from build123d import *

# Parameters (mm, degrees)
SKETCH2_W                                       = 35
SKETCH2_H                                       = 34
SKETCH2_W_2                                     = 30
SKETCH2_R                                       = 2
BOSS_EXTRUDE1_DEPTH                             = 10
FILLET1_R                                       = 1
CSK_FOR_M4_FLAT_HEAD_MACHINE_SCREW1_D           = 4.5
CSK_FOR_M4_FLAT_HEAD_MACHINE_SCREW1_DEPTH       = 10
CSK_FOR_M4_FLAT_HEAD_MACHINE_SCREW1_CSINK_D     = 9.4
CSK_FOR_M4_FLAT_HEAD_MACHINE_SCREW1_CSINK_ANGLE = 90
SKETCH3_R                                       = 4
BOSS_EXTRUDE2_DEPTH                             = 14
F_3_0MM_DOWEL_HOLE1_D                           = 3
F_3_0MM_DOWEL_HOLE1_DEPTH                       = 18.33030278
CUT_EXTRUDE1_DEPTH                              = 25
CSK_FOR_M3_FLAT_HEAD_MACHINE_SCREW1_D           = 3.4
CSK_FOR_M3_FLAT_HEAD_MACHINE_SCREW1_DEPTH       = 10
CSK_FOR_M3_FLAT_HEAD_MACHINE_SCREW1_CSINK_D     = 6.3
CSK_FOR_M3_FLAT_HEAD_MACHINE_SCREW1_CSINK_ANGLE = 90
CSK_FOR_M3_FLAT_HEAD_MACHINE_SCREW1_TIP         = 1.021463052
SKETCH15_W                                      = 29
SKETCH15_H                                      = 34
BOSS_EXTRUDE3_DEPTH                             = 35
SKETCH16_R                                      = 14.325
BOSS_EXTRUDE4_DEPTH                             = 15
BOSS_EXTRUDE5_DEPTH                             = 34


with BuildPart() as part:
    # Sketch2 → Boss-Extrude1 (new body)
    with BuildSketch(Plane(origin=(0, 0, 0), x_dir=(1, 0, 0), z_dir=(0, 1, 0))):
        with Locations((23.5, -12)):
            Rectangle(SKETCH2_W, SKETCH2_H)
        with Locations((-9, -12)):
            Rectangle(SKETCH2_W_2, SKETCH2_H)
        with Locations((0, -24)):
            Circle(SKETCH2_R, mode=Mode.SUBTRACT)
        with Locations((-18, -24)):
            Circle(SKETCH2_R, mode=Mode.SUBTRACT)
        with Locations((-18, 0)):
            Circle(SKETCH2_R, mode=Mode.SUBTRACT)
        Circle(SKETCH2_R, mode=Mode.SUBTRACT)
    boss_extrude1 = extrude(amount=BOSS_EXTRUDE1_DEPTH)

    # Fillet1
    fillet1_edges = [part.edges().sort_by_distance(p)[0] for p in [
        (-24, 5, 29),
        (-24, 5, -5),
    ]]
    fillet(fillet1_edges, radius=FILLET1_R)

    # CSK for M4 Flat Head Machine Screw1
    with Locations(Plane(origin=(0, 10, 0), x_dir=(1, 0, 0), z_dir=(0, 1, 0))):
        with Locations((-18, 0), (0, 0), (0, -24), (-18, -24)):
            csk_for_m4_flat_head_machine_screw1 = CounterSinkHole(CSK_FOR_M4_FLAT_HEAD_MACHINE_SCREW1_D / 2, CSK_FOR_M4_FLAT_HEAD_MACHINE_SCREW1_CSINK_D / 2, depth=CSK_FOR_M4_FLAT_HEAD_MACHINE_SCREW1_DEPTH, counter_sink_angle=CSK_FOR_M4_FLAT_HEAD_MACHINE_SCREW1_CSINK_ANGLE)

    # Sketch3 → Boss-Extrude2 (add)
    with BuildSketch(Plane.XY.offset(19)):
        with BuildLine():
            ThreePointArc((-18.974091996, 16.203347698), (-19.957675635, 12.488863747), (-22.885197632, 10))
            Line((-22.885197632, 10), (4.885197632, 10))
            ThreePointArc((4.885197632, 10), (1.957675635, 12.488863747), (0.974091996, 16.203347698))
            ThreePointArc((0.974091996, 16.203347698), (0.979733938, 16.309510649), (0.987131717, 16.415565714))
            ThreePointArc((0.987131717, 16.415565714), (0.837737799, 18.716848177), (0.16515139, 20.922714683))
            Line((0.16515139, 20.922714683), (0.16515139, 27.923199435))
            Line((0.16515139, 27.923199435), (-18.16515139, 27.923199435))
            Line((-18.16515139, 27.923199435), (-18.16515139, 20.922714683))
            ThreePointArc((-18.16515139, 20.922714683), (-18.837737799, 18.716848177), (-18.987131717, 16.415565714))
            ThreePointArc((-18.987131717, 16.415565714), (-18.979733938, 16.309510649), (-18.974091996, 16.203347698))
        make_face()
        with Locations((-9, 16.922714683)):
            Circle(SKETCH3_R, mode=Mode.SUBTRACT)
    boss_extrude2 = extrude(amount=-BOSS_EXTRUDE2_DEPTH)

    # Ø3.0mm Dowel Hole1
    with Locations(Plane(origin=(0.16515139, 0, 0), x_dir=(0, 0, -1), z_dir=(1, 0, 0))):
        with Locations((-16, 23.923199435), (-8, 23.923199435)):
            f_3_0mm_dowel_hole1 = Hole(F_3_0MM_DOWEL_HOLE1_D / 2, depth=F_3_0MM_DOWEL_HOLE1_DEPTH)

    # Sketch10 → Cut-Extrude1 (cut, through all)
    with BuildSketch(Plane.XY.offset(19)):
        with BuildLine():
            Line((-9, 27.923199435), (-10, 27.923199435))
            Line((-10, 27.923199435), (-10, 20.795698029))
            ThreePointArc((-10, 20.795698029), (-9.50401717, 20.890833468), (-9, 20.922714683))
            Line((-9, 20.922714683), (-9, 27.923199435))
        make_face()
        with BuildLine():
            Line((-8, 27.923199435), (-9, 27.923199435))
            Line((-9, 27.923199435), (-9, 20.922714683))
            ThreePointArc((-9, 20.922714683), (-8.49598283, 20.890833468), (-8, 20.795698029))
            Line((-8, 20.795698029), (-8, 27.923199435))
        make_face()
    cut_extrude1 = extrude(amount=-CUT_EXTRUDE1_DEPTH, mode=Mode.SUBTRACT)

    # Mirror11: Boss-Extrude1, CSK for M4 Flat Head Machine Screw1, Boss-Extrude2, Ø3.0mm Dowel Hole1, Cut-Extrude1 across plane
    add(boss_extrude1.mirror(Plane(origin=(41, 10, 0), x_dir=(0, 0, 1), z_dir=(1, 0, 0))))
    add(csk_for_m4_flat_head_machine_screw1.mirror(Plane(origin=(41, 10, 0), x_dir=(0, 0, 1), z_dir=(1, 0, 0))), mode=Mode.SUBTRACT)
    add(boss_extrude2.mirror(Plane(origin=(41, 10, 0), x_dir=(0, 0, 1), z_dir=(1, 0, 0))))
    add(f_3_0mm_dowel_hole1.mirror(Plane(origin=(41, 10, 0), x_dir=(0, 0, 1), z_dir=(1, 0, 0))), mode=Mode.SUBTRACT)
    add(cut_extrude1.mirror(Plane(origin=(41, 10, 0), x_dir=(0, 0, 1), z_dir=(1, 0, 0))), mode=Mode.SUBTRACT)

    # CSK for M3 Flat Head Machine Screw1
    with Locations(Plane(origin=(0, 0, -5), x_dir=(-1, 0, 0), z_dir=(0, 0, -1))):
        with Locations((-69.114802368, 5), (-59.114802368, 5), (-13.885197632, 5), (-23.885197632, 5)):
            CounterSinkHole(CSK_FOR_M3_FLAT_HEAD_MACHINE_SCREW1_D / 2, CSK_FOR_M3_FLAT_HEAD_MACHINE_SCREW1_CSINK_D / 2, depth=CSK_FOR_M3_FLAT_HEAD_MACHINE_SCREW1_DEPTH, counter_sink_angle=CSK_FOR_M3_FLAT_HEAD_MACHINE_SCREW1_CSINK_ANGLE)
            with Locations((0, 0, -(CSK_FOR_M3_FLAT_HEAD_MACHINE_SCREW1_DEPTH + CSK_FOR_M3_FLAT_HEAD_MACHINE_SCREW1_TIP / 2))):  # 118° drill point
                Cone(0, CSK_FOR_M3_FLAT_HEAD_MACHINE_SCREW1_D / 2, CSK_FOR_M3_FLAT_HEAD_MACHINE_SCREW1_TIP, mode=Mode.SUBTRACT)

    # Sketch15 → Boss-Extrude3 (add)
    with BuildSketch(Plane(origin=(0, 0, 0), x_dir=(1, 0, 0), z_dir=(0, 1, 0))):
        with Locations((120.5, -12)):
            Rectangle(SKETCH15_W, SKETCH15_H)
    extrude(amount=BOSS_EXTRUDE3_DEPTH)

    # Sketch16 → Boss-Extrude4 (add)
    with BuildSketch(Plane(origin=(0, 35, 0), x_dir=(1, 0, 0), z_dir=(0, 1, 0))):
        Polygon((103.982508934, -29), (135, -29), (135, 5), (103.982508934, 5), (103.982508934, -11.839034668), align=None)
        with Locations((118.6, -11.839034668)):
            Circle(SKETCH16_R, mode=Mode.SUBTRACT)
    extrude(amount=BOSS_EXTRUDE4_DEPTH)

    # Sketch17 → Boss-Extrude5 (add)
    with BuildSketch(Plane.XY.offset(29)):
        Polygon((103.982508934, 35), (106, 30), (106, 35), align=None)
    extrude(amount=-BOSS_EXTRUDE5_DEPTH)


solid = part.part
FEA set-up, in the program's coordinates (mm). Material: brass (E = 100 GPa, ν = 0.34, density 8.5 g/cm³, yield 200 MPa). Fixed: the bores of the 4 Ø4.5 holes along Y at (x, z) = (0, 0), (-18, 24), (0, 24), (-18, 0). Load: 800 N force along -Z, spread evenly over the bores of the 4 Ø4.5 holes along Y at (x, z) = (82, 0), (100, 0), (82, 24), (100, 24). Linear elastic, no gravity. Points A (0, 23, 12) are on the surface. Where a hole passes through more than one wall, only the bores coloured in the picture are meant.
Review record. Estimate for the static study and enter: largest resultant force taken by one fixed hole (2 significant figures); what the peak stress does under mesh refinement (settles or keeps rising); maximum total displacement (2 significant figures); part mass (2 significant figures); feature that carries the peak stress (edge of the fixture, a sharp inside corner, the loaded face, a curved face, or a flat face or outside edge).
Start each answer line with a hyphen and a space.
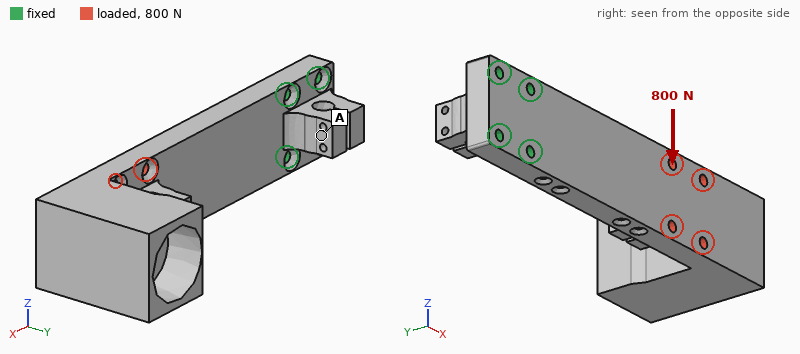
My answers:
- 2.7 kN
- keeps rising
- 0.13 mm
- 770 g
- edge of the fixture
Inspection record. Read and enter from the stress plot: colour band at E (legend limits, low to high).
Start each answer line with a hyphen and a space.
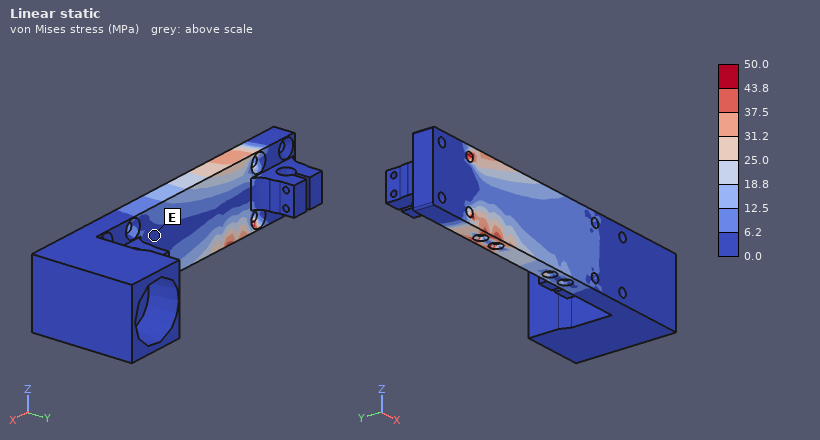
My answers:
- 0.0 to 6.2 MPa
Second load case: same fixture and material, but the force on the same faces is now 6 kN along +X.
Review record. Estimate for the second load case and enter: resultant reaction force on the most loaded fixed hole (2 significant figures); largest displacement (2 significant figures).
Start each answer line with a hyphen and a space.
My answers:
- 2.6 kN
- 0.23 mm
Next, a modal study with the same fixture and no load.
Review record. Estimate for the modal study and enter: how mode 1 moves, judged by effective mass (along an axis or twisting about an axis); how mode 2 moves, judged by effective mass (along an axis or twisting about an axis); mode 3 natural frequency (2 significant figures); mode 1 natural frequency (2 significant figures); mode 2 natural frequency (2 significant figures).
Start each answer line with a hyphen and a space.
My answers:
- along Y
- along Z
- 1000 Hz
- 170 Hz
- 470 Hz
